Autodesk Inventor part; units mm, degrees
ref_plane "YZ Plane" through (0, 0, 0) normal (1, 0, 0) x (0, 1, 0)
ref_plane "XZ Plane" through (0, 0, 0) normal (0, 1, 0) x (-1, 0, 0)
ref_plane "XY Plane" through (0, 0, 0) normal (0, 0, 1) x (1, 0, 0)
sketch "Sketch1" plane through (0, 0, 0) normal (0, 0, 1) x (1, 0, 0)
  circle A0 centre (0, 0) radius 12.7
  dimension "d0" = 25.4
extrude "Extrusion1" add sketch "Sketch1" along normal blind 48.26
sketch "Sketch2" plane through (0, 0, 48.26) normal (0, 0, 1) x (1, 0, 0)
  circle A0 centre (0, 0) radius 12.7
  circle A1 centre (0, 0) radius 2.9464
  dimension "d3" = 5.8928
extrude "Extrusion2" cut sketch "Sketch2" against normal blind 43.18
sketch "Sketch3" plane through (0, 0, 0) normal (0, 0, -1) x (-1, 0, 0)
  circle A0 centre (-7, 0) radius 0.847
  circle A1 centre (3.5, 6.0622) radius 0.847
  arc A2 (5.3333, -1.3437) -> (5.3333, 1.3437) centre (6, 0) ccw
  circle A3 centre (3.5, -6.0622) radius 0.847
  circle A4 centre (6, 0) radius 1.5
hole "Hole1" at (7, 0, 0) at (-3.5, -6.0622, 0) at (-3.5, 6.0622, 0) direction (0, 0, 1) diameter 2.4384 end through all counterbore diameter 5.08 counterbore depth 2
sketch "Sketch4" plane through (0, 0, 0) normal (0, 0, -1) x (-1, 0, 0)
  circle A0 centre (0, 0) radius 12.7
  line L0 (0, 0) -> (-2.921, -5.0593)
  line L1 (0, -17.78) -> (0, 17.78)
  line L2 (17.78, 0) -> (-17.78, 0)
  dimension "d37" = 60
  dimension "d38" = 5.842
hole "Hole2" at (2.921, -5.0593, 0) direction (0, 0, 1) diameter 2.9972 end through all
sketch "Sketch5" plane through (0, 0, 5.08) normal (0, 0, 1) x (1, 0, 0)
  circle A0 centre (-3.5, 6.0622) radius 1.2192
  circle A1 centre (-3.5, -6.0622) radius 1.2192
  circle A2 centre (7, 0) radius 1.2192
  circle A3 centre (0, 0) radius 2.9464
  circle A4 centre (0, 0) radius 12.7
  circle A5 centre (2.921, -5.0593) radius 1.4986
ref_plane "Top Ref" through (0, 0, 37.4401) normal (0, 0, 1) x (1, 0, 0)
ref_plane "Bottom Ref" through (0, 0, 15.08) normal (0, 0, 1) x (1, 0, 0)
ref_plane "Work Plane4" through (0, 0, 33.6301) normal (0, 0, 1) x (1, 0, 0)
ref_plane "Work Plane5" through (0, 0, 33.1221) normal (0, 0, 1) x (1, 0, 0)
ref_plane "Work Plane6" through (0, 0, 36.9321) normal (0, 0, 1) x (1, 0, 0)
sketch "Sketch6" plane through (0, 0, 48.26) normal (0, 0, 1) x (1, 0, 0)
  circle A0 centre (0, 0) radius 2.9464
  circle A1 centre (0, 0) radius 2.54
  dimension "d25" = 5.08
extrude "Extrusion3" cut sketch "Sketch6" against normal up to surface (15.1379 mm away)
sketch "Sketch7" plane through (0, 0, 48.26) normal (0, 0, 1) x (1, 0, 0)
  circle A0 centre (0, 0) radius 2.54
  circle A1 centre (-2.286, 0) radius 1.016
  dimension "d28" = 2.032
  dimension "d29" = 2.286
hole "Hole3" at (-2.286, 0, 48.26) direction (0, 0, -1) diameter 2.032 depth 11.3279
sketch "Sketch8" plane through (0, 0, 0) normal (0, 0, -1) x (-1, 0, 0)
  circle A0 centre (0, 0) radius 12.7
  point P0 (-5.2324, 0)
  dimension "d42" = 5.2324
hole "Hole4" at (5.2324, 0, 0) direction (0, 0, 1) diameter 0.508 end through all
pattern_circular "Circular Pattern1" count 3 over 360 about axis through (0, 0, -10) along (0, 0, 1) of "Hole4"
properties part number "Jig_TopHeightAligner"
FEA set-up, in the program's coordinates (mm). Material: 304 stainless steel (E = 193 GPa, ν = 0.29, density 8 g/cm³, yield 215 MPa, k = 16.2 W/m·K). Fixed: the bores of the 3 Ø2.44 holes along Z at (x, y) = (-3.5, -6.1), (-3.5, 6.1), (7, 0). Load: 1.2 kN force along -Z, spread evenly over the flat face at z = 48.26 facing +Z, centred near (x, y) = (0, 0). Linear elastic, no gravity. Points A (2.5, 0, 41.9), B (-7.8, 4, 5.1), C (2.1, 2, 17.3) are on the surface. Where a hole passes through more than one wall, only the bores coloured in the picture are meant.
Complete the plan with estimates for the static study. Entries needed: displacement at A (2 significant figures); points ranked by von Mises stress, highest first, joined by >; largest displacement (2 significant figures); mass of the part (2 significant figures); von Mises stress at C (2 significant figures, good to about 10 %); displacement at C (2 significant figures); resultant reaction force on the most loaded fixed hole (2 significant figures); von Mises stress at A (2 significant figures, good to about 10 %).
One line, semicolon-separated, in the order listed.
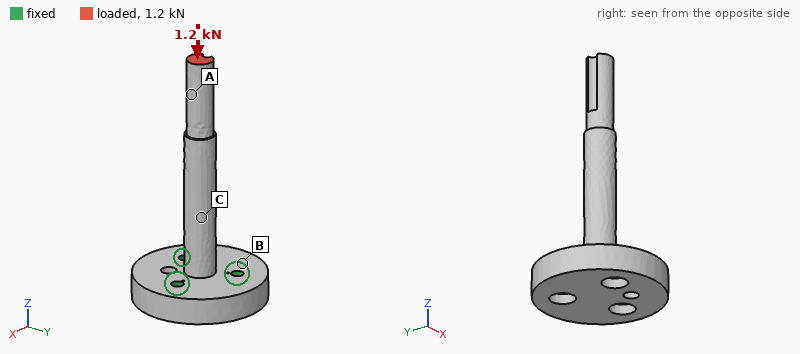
21 µm; A > C > B; 27 µm; 27 g; 53 MPa; 5.5 µm; 430 N; 66 MPa
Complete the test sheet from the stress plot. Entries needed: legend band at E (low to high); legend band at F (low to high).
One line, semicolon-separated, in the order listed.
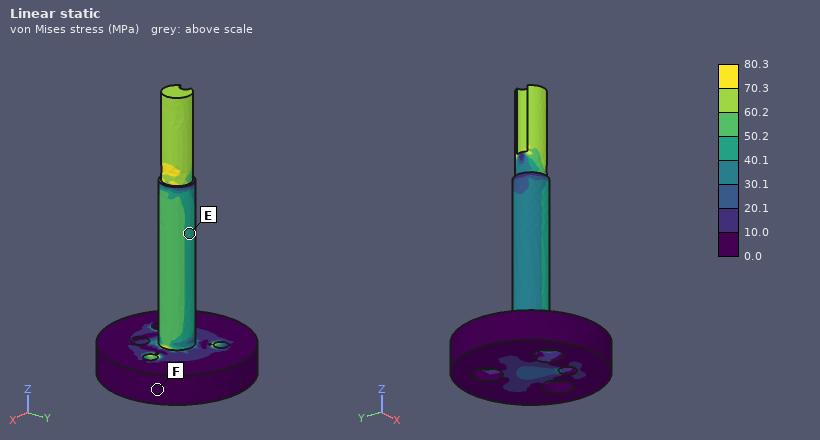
40.1 to 50.2 MPa; 0.0 to 10.0 MPa
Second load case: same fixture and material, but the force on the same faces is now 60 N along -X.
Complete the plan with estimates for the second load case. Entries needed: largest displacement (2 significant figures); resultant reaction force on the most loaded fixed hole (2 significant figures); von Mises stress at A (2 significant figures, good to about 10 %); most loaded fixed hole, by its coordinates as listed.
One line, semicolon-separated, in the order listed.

0.17 mm; 240 N; 37 MPa; (7, 0)
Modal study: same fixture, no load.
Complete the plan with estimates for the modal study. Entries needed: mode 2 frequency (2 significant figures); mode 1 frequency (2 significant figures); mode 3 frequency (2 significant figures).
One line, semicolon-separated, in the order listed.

2300 Hz; 2300 Hz; 12 kHz
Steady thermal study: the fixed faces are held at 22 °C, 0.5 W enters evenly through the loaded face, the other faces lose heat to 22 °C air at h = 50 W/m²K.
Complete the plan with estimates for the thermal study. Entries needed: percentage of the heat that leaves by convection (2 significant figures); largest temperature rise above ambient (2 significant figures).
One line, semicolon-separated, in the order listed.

78 %; 29 K
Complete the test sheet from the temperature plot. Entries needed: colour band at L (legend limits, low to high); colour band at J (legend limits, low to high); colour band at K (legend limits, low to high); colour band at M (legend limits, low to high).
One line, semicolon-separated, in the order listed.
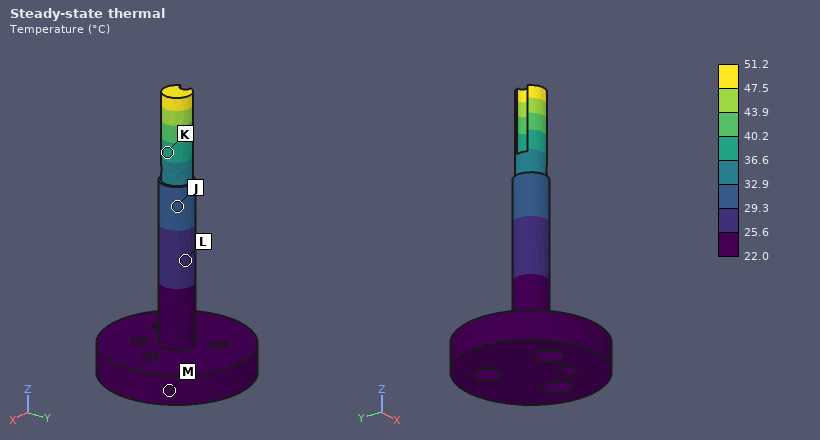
25.6 to 29.3 °C; 29.3 to 32.9 °C; 36.6 to 40.2 °C; 22.0 to 25.6 °C
